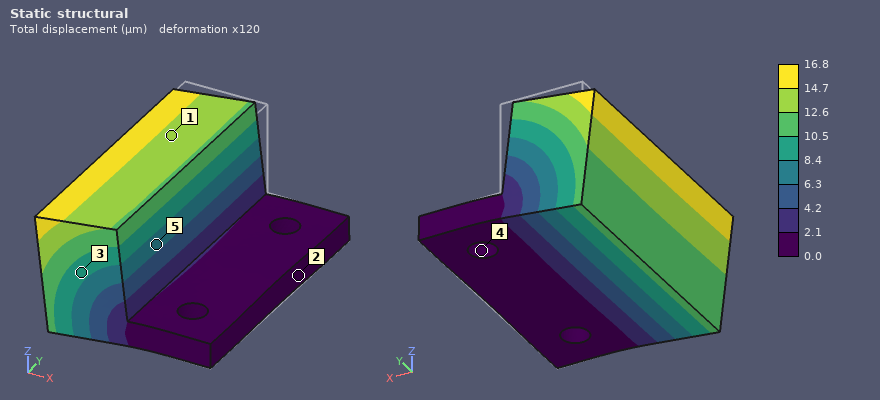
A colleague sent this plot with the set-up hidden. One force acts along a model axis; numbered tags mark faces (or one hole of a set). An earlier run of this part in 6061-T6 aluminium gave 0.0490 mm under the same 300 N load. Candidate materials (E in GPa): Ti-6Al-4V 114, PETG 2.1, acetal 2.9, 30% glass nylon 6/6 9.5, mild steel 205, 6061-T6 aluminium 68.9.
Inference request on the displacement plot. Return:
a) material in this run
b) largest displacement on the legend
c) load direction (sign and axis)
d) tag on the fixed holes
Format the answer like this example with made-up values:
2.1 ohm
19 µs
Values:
mild steel
16.8 µm
-X
4
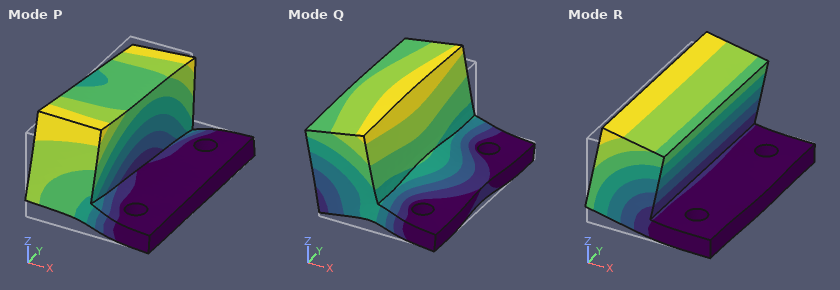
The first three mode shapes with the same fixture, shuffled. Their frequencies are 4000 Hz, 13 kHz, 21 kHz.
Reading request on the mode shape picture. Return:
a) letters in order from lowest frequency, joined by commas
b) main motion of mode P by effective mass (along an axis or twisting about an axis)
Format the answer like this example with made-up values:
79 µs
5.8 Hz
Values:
R, P, Q
along Y
